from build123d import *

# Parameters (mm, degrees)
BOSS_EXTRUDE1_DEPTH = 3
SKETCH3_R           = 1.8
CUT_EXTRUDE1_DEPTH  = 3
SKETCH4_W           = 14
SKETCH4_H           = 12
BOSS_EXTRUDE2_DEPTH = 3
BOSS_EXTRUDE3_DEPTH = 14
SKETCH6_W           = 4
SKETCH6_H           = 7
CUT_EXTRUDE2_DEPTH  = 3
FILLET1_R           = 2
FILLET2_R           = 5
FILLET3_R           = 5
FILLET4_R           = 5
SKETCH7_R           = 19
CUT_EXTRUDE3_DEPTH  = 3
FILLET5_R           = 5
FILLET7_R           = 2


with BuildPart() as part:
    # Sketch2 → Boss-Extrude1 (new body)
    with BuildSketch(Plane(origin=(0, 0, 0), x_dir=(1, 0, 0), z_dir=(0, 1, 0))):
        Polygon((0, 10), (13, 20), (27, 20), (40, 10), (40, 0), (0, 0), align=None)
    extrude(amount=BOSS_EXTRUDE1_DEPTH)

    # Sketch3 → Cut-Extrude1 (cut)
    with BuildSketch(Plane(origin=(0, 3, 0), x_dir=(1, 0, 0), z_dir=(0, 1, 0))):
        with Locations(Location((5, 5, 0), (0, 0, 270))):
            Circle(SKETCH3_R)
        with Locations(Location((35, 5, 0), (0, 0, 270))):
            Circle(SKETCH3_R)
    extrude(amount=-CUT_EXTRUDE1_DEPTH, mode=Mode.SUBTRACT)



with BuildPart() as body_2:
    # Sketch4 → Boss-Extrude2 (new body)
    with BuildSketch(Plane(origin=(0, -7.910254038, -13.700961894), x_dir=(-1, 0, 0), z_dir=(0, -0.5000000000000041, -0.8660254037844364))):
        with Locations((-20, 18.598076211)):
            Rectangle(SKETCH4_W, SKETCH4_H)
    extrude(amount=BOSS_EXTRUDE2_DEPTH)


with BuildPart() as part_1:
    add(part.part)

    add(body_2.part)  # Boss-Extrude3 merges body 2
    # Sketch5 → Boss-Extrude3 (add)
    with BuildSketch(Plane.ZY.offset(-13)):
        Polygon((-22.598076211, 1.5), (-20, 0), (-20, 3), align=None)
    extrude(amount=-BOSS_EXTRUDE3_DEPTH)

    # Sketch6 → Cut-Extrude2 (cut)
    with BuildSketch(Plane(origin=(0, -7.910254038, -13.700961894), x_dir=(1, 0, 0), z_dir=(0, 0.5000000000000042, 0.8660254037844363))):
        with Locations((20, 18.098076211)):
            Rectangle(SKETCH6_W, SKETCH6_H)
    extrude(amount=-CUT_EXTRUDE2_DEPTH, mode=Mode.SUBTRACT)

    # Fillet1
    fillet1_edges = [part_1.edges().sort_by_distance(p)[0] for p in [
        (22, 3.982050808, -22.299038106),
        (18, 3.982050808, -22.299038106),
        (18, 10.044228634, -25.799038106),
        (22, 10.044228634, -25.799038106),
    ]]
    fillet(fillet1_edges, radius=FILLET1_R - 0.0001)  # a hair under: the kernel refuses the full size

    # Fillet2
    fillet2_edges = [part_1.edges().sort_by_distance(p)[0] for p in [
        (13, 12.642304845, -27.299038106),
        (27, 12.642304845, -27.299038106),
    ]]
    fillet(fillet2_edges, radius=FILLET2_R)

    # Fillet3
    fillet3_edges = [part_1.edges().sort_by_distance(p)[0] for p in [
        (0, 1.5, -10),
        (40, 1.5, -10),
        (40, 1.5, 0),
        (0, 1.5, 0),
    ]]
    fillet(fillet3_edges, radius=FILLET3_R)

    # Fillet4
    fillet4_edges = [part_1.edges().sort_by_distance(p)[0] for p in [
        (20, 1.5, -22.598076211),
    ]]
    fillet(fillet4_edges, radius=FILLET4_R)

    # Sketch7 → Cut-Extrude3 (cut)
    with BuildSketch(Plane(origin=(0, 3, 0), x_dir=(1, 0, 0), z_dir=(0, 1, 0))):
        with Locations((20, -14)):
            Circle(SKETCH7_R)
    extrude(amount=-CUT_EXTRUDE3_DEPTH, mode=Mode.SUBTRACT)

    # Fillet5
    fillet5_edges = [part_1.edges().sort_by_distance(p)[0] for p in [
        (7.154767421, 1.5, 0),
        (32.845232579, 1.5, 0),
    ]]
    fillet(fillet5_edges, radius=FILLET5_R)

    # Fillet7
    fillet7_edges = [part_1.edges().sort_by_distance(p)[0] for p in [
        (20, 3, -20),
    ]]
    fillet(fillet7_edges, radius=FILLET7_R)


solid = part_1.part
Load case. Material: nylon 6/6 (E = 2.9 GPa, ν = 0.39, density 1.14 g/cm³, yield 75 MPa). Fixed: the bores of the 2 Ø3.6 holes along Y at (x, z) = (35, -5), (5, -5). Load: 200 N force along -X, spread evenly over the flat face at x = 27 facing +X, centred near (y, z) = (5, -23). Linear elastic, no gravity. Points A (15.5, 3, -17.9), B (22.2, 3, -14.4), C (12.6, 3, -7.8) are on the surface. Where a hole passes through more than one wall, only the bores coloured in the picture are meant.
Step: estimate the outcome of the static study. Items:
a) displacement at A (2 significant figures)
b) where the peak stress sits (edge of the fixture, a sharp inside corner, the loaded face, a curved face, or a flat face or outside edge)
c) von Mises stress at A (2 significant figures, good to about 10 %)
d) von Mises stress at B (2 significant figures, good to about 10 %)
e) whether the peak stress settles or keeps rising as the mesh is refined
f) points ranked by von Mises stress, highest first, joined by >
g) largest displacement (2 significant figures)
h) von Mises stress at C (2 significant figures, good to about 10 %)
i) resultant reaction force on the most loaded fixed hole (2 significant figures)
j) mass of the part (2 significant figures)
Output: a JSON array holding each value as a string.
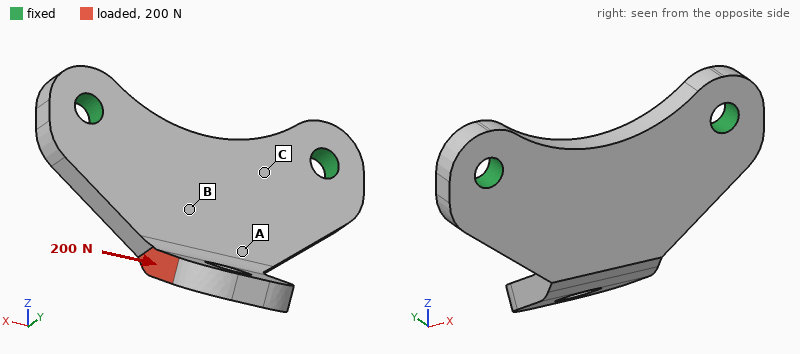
["0.11 mm", "a sharp inside corner", "20 MPa", "13 MPa", "keeps rising", "A > B > C", "0.44 mm", "5.9 MPa", "160 N", "2.4 g"]
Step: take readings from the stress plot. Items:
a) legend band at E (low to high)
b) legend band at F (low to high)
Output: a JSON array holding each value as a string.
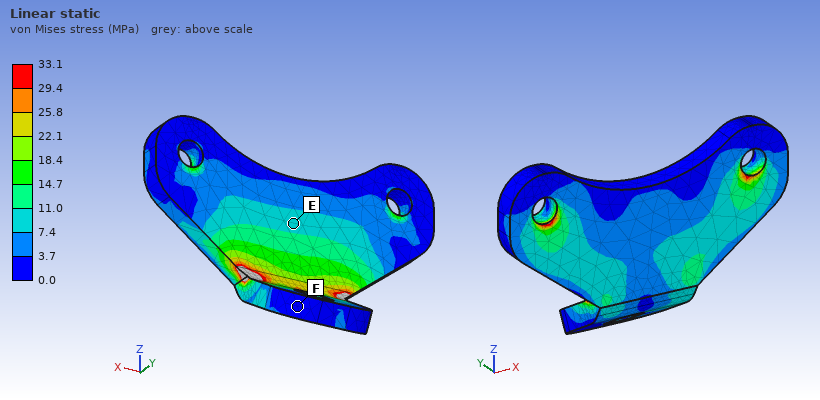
["7.4 to 11.0 MPa", "0.0 to 3.7 MPa"]
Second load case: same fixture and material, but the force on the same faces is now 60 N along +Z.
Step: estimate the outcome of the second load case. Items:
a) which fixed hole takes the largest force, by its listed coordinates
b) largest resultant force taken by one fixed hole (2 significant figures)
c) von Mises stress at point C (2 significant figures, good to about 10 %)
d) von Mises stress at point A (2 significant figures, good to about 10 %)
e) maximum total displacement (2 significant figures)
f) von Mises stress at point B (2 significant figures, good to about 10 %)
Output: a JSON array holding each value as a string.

["(35, -5)", "50 N", "4.5 MPa", "5.2 MPa", "0.53 mm", "6.5 MPa"]
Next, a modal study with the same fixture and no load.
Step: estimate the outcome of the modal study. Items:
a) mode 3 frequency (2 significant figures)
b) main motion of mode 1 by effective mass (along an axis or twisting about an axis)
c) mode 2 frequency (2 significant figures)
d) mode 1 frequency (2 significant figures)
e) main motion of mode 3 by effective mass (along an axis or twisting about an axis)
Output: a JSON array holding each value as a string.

["4100 Hz", "along Y", "3700 Hz", "1300 Hz", "along Y"]
